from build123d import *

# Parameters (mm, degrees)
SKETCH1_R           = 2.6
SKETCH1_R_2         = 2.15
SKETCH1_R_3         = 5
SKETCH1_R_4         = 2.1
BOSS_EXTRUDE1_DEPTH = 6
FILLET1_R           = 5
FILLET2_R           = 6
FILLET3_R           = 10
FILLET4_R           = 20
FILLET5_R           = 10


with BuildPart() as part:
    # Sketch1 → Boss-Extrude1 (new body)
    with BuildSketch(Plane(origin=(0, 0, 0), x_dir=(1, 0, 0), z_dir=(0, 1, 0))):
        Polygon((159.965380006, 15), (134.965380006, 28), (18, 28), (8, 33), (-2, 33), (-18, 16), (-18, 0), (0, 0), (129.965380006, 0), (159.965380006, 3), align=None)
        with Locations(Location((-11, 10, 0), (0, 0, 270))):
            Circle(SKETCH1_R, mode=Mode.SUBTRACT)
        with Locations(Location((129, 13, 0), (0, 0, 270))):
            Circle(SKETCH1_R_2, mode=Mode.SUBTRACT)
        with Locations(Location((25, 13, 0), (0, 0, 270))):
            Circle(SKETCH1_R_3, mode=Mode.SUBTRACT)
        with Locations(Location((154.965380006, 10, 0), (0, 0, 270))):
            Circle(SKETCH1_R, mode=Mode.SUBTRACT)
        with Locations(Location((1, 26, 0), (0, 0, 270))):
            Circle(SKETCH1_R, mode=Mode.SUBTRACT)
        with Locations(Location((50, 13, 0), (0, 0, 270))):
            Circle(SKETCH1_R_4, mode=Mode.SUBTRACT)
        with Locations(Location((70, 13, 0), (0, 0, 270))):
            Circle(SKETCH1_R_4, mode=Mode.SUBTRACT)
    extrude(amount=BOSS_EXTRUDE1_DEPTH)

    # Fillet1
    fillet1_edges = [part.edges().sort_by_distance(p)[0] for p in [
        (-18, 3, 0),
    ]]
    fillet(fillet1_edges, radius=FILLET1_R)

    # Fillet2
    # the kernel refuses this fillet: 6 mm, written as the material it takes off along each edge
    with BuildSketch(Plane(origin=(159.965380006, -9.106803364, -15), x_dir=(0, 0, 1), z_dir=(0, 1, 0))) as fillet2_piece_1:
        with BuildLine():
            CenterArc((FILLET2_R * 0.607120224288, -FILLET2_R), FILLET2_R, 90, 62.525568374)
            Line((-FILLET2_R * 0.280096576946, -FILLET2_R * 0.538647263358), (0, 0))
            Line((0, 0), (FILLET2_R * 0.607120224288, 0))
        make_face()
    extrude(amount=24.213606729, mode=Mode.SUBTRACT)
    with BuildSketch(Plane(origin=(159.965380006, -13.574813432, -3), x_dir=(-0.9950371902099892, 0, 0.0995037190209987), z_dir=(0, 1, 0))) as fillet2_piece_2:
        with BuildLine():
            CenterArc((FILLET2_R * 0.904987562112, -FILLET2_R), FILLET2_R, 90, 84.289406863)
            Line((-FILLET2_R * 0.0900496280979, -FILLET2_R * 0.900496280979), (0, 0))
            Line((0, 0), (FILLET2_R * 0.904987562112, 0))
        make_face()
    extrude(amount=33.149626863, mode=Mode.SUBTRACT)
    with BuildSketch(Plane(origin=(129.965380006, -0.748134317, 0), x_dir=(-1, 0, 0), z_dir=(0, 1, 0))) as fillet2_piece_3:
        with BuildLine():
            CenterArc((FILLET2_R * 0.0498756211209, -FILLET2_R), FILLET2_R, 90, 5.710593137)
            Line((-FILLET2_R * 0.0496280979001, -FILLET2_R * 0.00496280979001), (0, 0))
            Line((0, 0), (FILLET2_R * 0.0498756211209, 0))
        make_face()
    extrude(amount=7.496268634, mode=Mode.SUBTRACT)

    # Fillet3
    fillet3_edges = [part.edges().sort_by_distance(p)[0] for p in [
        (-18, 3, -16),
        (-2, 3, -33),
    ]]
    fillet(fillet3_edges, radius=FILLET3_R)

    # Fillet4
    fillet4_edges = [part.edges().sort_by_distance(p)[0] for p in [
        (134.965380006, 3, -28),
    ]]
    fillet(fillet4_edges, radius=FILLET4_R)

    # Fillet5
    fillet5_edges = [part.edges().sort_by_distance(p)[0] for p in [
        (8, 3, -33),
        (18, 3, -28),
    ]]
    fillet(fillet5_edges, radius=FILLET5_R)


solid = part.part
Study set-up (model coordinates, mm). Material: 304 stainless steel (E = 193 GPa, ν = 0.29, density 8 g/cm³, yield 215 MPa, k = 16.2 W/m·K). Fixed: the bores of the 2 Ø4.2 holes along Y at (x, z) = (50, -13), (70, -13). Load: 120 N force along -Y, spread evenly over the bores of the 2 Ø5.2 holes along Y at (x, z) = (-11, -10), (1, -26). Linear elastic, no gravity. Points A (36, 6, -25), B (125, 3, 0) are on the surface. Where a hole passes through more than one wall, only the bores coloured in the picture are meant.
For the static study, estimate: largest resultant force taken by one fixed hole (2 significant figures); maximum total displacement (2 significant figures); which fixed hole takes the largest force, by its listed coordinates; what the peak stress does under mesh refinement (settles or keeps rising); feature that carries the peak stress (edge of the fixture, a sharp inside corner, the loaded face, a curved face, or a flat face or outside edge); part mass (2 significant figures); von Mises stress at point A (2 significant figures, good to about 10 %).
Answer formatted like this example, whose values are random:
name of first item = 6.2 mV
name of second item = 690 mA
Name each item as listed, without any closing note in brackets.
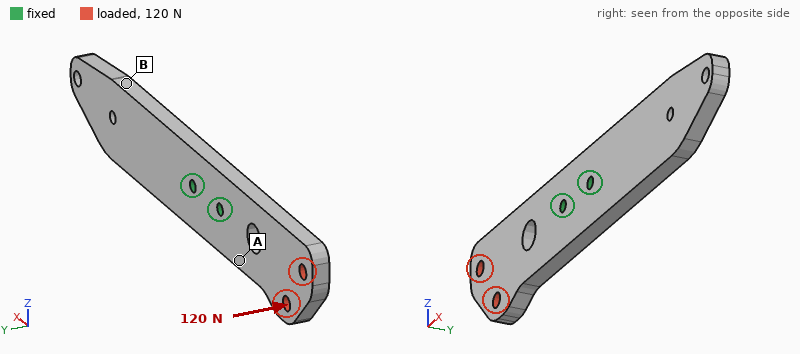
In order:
largest resultant force taken by one fixed hole = 250 N
maximum total displacement = 0.11 mm
which fixed hole takes the largest force, by its listed coordinates = (50, -13)
what the peak stress does under mesh refinement = keeps rising
feature that carries the peak stress = edge of the fixture
part mass = 220 g
von Mises stress at point A = 32 MPa
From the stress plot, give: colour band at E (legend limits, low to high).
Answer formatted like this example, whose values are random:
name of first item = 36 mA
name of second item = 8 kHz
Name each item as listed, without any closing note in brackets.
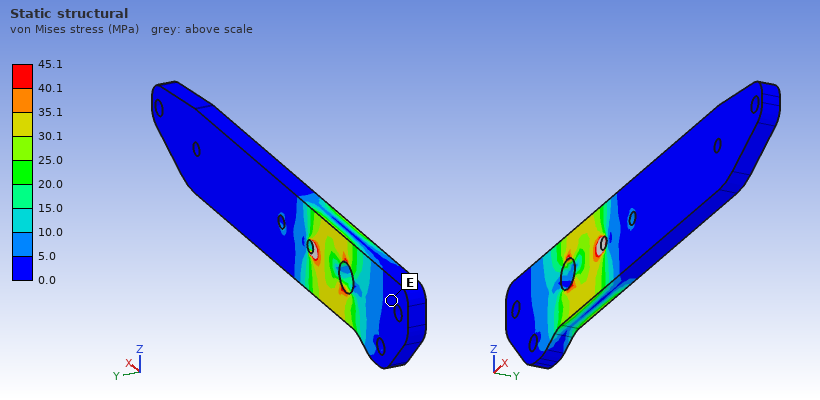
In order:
colour band at E = 0.0 to 5.0 MPa
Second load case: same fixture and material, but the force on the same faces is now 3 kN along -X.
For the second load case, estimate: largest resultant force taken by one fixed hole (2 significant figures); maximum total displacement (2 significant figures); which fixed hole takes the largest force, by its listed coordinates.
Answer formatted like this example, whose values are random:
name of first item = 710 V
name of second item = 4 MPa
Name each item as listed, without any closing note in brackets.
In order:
largest resultant force taken by one fixed hole = 2.3 kN
maximum total displacement = 19 µm
which fixed hole takes the largest force, by its listed coordinates = (50, -13)
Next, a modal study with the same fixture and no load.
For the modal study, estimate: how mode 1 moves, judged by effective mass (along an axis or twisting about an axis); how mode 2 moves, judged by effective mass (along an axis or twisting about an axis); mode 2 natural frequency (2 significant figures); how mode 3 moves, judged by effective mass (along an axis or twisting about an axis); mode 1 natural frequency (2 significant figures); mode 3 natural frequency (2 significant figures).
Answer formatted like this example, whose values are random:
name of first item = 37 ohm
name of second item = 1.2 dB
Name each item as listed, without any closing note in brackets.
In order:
how mode 1 moves, judged by effective mass = along Y
how mode 2 moves, judged by effective mass = along Y
mode 2 natural frequency = 1000 Hz
how mode 3 moves, judged by effective mass = along Z
mode 1 natural frequency = 690 Hz
mode 3 natural frequency = 2300 Hz
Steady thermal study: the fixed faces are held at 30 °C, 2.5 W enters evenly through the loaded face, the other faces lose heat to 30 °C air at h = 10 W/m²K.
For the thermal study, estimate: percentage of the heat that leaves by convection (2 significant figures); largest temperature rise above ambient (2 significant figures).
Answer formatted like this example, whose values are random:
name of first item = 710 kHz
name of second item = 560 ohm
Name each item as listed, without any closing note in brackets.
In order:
percentage of the heat that leaves by convection = 43 %
largest temperature rise above ambient = 40 K
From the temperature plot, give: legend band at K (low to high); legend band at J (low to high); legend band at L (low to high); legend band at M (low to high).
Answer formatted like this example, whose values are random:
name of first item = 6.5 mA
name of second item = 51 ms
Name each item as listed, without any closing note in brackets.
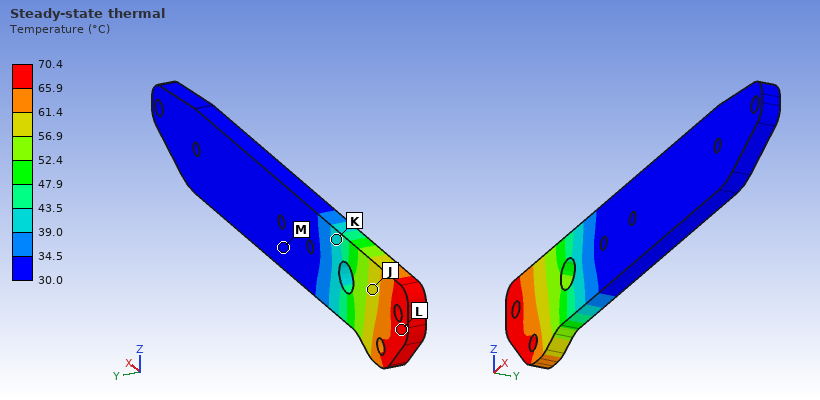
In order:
legend band at K = 39.0 to 43.5 °C
legend band at J = 56.9 to 61.4 °C
legend band at L = 65.9 to 70.4 °C
legend band at M = 30.0 to 34.5 °C
